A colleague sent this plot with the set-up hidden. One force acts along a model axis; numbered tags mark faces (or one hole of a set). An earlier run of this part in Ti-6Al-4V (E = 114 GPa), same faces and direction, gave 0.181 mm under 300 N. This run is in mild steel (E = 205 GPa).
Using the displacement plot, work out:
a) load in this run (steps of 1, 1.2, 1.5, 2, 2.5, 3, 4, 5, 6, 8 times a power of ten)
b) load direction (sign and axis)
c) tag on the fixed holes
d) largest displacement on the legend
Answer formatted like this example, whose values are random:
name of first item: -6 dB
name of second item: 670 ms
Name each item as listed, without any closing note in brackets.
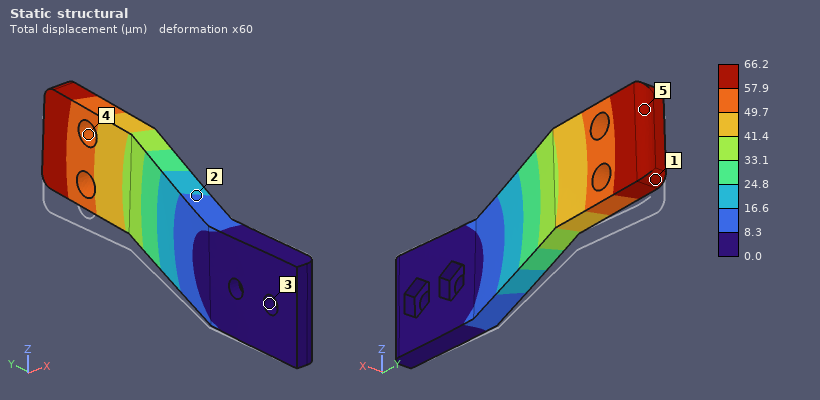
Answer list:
load in this run: 200 N
load direction: +Z
tag on the fixed holes: 3
largest displacement on the legend: 66.2 µm
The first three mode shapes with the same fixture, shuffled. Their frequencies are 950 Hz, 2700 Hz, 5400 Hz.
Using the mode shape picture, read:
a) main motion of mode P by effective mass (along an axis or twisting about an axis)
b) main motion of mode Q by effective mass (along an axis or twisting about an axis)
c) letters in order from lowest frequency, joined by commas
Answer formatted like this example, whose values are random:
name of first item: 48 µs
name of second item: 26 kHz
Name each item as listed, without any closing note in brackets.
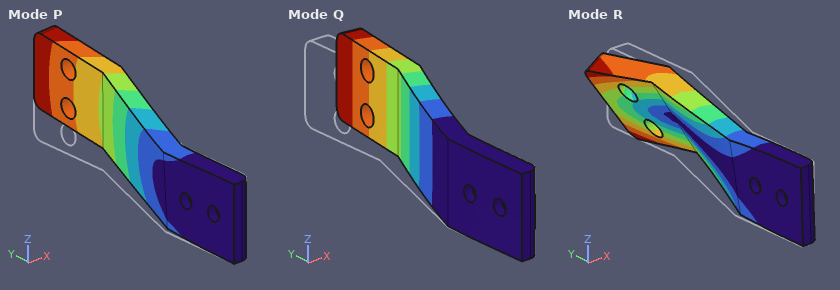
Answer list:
main motion of mode P by effective mass: along Z
main motion of mode Q by effective mass: along X
letters in order from lowest frequency, joined by commas: Q, P, R
